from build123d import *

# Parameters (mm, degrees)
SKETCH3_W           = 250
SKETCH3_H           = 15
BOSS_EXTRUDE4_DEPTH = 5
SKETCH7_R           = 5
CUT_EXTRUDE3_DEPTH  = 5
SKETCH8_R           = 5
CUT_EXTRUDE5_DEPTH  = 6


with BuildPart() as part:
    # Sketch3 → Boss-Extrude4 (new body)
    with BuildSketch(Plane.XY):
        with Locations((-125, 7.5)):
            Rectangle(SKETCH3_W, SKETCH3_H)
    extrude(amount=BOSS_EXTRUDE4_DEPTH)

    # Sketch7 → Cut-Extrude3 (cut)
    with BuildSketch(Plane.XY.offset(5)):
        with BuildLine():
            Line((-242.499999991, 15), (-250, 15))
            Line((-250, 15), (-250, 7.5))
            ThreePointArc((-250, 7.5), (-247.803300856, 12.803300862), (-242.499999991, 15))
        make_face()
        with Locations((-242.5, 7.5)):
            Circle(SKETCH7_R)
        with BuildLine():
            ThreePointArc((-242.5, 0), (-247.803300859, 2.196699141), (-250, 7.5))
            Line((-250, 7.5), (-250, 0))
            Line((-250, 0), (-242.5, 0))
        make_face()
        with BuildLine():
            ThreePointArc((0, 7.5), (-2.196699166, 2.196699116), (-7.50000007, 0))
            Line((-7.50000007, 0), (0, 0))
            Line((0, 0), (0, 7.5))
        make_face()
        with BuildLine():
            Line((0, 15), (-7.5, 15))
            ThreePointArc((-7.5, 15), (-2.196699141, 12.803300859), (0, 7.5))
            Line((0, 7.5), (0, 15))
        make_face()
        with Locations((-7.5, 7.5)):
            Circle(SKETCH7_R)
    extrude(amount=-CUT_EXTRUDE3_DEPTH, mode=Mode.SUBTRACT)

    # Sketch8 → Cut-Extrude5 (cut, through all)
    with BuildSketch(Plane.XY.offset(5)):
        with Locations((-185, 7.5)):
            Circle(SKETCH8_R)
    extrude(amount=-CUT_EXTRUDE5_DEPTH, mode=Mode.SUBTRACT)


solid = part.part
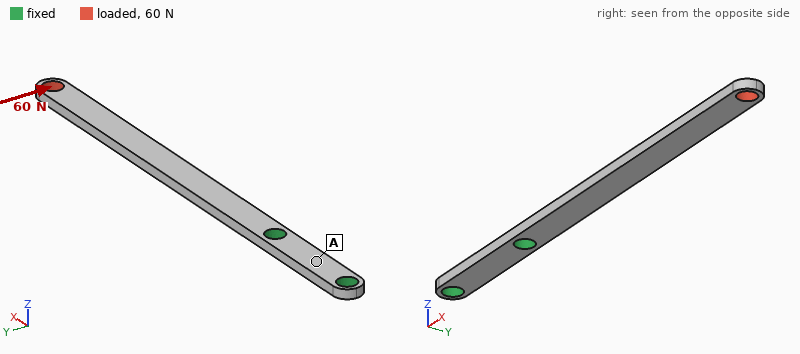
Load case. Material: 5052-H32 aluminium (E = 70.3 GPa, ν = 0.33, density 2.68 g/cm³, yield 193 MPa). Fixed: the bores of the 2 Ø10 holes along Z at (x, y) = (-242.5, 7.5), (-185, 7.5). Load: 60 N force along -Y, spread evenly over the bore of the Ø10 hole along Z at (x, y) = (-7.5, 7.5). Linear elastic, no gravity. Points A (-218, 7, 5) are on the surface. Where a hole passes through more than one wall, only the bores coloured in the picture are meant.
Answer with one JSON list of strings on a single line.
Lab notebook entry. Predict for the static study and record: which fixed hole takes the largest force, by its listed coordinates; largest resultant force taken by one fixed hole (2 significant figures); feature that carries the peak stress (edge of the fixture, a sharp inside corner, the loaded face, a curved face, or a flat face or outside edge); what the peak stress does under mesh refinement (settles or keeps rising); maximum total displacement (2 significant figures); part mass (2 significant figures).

["(-185, 7.5)", "66 N", "edge of the fixture", "keeps rising", "1.2 mm", "46 g"]
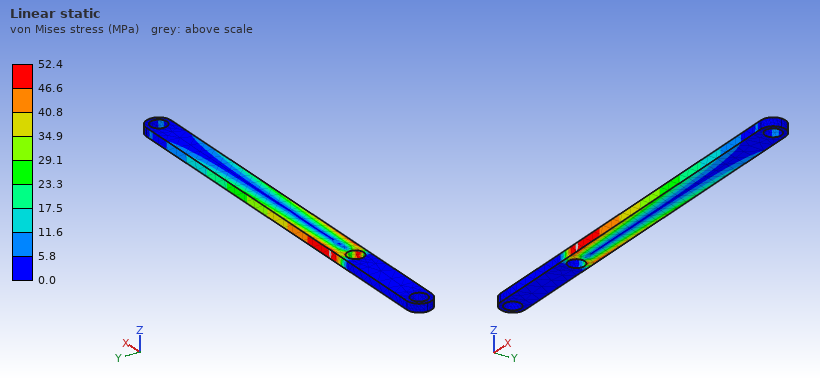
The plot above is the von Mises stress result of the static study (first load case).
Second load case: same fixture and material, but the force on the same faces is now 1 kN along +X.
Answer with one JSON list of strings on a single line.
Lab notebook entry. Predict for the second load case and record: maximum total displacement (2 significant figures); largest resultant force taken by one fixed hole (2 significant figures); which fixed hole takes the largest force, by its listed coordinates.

["42 µm", "1000 N", "(-185, 7.5)"]
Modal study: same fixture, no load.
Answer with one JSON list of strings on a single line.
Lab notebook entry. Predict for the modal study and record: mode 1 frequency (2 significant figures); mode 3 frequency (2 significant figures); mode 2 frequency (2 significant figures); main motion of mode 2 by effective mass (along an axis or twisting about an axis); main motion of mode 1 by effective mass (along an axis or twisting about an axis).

["140 Hz", "840 Hz", "390 Hz", "along Y", "along Z"]
